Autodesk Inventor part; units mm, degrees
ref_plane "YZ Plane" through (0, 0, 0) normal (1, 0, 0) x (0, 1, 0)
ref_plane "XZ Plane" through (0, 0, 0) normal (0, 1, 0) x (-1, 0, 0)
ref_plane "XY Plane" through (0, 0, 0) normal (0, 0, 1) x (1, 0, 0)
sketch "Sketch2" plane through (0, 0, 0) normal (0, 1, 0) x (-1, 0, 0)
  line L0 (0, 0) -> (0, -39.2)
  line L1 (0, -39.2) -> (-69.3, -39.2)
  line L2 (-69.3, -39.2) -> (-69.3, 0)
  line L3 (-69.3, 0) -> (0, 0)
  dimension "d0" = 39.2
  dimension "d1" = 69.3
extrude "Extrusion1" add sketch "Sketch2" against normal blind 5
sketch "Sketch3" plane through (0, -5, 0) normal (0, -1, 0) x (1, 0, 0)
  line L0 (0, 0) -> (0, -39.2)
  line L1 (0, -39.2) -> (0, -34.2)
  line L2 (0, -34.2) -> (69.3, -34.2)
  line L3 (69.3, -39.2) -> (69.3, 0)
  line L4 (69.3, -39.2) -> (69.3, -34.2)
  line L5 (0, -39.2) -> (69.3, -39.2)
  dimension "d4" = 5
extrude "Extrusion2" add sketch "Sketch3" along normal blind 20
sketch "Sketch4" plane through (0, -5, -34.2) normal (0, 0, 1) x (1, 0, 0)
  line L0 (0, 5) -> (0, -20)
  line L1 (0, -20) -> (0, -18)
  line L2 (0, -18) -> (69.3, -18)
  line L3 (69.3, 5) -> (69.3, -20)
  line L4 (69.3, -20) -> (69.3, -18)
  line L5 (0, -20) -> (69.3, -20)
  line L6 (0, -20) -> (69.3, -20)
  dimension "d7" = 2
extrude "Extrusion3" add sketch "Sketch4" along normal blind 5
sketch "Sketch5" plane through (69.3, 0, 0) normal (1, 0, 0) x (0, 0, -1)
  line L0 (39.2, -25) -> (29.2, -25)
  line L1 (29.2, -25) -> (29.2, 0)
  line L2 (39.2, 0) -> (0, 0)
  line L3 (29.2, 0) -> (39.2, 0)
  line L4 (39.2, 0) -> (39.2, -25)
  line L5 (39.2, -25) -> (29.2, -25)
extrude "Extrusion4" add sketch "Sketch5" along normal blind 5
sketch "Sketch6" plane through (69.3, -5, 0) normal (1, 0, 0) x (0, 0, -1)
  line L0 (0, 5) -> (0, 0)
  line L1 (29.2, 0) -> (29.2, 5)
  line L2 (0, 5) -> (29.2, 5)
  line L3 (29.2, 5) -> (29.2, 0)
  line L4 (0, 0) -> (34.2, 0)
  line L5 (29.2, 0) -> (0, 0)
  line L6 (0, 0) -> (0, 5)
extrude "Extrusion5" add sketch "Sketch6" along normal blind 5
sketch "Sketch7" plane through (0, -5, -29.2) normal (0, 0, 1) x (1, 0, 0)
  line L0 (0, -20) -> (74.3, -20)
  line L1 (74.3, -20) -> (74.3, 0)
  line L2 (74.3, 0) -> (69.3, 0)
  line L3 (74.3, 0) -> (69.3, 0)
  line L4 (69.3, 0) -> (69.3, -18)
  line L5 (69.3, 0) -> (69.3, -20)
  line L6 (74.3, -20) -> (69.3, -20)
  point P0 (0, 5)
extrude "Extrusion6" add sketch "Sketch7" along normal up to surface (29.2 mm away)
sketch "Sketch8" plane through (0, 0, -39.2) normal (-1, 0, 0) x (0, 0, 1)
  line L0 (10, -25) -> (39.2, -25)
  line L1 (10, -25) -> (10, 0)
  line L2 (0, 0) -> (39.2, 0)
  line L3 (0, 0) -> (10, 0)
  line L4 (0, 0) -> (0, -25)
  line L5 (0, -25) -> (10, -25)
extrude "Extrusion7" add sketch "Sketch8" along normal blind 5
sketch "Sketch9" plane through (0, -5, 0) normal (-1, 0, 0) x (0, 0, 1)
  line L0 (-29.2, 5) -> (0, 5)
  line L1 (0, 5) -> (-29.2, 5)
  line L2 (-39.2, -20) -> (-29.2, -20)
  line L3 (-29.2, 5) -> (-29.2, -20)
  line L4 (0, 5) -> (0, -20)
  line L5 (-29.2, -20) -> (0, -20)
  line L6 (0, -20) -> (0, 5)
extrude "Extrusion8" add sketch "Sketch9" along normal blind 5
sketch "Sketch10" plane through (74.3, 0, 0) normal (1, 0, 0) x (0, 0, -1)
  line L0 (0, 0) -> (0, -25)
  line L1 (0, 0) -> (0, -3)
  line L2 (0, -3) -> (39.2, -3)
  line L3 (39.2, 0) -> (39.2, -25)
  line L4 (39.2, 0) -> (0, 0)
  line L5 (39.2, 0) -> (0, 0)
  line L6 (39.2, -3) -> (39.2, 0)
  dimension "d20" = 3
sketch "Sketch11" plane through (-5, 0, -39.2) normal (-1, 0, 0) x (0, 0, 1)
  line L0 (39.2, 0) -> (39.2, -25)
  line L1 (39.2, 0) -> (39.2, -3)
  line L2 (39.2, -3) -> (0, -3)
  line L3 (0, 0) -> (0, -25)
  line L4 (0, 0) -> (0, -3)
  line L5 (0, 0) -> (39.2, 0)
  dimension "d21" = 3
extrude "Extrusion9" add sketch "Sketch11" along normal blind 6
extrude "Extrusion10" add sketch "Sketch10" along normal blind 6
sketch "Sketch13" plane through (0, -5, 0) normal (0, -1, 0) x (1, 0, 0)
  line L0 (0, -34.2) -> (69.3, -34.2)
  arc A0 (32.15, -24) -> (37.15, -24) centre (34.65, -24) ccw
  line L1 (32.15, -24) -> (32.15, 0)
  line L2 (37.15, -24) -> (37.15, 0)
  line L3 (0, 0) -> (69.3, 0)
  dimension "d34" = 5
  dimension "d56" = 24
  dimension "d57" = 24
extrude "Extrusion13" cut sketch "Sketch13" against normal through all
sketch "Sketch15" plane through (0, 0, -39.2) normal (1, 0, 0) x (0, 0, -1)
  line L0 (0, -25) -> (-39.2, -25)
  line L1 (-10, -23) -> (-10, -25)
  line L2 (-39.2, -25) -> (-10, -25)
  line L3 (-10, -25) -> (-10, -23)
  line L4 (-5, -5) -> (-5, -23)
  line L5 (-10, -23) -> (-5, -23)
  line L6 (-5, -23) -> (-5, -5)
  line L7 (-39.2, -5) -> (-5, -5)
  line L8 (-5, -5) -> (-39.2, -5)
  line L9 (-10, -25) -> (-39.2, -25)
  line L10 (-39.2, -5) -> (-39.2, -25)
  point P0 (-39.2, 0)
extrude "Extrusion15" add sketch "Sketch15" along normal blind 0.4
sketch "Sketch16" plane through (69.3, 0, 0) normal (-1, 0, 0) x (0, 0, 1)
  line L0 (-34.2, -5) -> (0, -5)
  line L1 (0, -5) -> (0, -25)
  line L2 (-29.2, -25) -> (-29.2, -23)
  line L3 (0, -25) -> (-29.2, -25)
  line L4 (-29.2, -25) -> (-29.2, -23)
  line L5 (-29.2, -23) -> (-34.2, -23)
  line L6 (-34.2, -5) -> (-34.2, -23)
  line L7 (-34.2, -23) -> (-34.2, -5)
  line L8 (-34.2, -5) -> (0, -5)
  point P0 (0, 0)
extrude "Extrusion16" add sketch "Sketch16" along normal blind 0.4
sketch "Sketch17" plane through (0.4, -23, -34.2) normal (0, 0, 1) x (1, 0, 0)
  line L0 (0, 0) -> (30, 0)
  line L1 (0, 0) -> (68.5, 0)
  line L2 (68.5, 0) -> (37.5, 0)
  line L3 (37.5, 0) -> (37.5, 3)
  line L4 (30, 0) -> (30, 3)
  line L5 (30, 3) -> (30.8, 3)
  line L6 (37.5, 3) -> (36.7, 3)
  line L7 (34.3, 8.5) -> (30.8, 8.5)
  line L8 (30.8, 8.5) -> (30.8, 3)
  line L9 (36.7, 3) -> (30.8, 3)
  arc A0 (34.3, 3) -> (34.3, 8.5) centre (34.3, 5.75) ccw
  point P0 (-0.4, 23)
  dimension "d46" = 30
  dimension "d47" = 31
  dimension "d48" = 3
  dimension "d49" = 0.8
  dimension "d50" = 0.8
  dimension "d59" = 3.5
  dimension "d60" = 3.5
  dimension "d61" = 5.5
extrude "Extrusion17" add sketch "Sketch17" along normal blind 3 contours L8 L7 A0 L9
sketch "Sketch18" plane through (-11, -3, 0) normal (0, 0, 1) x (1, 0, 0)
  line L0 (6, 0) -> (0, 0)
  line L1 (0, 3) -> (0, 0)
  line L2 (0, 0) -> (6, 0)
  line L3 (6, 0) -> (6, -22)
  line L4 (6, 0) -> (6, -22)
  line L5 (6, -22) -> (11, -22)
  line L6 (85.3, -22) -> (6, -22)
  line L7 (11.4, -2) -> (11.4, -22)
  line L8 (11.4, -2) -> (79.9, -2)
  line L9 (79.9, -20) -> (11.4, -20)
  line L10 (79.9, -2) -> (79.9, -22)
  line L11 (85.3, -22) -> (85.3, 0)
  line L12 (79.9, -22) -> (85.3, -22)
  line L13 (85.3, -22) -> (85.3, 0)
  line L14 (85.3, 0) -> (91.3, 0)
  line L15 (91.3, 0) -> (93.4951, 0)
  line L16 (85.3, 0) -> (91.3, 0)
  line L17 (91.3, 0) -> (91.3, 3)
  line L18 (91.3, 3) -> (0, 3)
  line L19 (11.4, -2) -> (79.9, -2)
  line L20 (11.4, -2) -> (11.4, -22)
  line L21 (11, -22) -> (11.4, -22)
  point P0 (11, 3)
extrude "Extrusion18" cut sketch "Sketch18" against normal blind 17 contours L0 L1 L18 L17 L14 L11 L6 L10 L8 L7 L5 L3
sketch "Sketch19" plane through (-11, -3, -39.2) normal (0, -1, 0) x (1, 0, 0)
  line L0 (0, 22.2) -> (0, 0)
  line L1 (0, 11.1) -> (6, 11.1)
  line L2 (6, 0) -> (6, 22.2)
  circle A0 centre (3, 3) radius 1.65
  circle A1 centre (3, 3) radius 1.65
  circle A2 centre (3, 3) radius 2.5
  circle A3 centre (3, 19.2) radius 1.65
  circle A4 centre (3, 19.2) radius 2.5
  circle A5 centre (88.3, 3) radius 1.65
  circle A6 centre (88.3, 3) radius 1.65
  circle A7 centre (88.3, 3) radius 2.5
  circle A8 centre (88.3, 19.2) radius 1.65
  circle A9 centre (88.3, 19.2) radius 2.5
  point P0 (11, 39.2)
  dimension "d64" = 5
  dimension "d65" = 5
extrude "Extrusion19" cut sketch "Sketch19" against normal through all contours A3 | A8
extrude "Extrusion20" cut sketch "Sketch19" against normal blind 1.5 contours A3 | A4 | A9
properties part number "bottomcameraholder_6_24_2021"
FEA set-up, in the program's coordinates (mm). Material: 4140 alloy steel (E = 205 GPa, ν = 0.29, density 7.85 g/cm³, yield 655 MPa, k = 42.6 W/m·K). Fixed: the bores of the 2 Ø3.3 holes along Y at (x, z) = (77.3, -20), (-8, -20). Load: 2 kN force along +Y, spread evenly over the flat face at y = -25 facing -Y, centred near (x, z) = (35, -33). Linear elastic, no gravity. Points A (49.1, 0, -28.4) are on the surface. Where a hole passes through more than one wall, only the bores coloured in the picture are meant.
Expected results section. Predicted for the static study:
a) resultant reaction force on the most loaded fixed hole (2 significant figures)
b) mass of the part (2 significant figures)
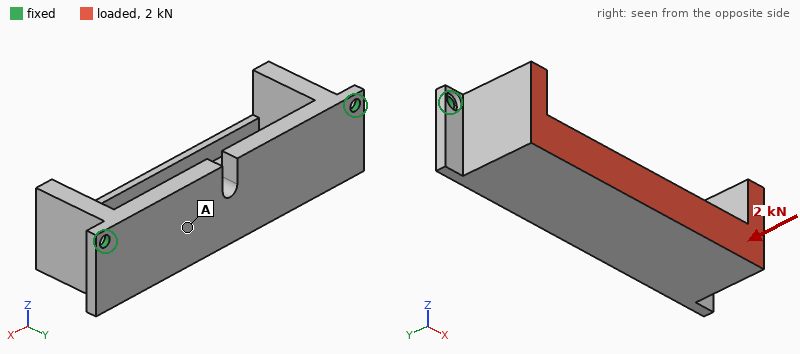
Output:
1.0 kN
170 g
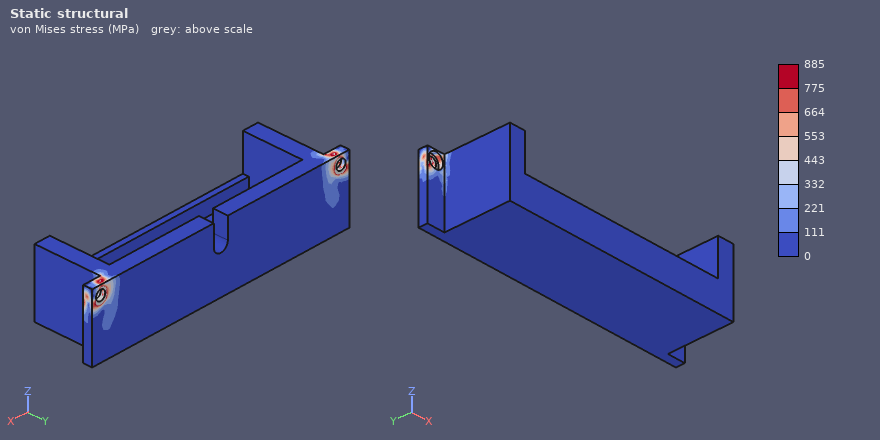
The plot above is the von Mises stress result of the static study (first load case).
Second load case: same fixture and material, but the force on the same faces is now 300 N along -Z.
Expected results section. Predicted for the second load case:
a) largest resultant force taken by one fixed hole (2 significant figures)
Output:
190 N
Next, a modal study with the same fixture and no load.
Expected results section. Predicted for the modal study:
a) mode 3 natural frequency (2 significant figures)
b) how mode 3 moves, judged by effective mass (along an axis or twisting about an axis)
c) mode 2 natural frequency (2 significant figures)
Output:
5400 Hz
along Y
3200 Hz
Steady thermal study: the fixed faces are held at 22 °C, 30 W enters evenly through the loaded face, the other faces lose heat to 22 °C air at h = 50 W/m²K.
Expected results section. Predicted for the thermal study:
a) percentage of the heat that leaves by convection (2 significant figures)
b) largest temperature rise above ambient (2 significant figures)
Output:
63 %
66 K
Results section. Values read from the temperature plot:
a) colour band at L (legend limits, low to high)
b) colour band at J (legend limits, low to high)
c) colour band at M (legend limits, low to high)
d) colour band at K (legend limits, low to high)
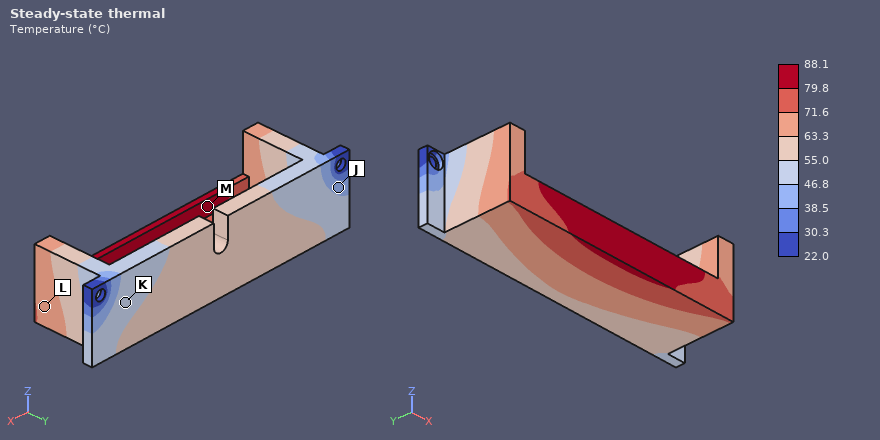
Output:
63.3 to 71.6 °C
38.5 to 46.8 °C
79.8 to 88.1 °C
46.8 to 55.0 °C
